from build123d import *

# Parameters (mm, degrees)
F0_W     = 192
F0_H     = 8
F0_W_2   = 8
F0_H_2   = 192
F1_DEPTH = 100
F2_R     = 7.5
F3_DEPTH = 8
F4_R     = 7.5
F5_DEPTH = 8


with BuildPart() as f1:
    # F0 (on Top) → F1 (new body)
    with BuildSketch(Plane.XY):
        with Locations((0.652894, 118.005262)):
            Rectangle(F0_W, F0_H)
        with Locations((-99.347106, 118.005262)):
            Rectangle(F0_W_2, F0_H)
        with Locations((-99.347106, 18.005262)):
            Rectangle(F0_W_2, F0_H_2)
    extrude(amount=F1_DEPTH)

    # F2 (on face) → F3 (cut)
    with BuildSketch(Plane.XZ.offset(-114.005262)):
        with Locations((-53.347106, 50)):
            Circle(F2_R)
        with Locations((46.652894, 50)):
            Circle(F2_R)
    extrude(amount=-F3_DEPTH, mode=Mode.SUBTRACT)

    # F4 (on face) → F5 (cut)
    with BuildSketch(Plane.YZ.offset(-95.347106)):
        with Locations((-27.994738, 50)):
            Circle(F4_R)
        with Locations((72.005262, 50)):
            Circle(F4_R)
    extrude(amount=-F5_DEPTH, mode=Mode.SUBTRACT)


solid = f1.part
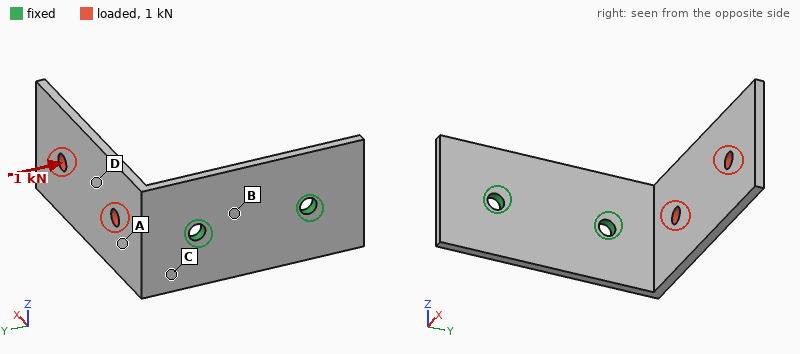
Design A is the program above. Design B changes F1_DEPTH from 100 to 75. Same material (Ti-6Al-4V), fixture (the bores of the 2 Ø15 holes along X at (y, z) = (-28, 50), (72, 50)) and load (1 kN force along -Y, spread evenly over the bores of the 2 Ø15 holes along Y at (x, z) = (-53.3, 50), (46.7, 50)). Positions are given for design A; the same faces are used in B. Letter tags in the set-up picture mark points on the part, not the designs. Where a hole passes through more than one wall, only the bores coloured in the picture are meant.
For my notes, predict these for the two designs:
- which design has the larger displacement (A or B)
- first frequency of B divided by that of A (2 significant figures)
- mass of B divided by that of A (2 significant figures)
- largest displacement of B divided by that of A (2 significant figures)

B
1.0
0.75
1.3
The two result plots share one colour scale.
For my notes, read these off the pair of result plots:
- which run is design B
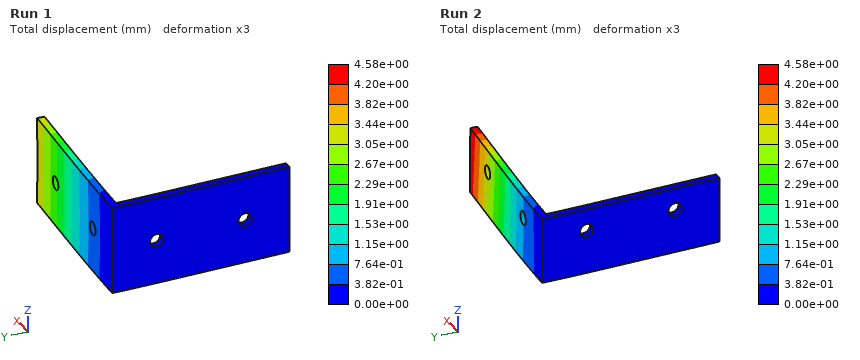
Run 2
